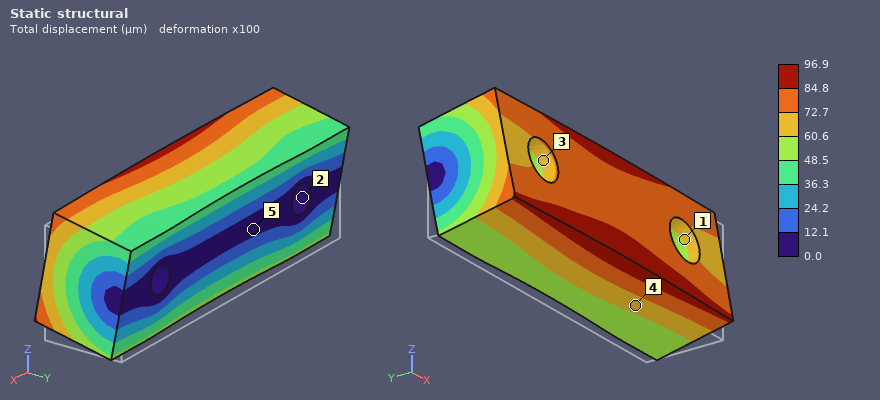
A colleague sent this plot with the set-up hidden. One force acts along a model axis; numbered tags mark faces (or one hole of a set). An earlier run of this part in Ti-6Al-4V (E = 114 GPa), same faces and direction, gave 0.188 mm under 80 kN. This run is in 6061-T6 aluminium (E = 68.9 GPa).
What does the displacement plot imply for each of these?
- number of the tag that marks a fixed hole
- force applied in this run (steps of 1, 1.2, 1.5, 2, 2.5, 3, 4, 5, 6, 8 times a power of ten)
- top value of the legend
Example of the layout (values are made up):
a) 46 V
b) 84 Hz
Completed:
a) 2
b) 25 kN
c) 96.9 µm
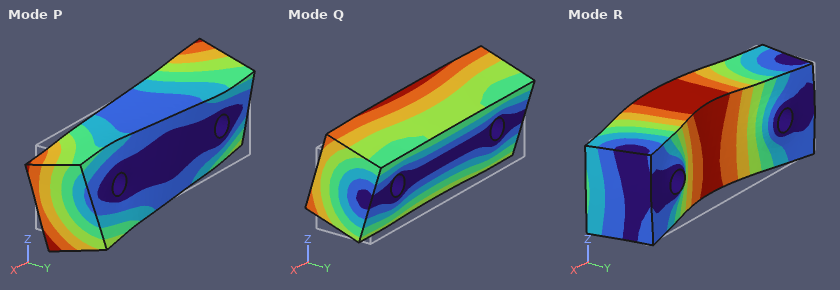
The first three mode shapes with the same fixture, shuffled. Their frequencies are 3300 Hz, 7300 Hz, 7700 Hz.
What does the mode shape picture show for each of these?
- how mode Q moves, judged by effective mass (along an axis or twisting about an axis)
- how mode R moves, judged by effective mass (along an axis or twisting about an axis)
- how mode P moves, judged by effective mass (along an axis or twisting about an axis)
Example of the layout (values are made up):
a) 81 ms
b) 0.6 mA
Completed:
a) along Z
b) along Y
c) twisting about Y
